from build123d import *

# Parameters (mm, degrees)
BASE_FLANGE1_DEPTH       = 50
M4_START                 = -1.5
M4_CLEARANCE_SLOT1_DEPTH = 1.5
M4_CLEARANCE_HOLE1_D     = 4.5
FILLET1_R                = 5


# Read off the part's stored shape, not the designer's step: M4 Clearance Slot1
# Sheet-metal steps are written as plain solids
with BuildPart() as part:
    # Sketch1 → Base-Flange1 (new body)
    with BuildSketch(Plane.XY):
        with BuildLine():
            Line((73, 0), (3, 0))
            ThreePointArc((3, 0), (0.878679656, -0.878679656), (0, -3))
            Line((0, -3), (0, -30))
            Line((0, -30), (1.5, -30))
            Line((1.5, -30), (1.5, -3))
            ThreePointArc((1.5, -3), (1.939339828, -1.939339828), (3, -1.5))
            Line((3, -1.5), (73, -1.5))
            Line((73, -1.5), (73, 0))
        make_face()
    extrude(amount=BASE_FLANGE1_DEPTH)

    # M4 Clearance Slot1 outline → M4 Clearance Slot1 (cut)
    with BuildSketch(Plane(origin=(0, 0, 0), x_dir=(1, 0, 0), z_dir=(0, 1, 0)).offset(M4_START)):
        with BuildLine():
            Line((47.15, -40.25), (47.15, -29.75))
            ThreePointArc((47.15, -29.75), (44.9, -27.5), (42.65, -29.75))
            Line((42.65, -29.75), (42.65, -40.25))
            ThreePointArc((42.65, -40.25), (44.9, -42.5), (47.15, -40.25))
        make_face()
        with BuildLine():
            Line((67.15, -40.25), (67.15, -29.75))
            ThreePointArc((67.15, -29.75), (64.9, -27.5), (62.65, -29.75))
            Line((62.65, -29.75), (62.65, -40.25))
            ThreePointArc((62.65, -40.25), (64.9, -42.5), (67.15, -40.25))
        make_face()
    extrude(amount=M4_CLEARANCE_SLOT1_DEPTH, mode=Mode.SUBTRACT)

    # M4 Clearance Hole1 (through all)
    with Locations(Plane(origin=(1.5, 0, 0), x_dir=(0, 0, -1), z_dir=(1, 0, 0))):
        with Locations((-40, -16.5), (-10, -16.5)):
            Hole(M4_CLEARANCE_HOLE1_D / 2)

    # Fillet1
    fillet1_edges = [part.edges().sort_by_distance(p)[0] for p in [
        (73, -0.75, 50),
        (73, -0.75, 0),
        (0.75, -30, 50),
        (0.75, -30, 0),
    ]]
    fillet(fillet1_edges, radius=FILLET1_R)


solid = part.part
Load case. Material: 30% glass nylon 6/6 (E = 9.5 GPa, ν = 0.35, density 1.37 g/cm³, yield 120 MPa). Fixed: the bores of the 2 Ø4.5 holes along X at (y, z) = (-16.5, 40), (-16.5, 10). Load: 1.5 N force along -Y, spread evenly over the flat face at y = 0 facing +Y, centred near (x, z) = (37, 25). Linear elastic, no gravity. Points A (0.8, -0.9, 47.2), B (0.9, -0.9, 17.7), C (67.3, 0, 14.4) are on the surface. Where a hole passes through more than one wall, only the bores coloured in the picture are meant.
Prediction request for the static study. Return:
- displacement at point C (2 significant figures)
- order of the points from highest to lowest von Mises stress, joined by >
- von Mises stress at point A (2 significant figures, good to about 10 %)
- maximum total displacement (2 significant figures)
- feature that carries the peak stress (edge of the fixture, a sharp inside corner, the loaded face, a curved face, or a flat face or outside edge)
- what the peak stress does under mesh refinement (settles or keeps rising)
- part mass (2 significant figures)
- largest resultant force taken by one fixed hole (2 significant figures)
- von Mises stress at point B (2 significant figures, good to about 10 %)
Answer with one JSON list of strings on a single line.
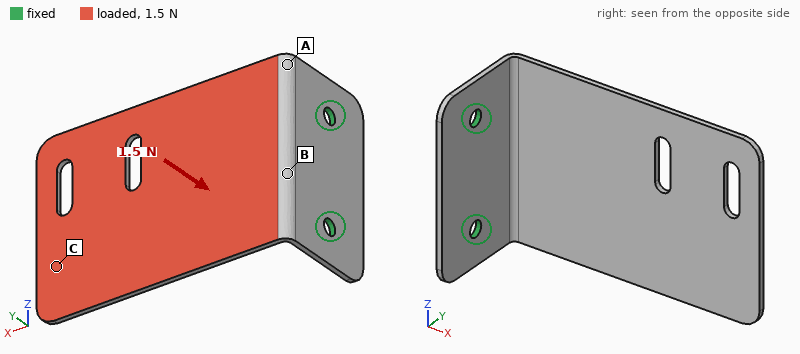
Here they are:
["0.81 mm", "B > A > C", "1.7 MPa", "0.89 mm", "edge of the fixture", "keeps rising", "10.0 g", "0.83 N", "2.2 MPa"]
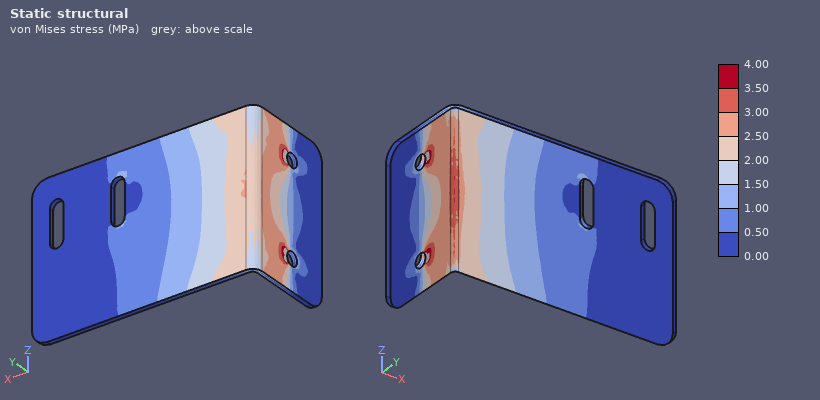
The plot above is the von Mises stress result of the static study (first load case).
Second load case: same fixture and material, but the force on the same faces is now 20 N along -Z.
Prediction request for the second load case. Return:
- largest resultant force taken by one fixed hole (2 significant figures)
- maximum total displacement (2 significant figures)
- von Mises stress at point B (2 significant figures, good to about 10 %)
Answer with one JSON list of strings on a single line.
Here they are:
["26 N", "1.00 mm", "8.0 MPa"]
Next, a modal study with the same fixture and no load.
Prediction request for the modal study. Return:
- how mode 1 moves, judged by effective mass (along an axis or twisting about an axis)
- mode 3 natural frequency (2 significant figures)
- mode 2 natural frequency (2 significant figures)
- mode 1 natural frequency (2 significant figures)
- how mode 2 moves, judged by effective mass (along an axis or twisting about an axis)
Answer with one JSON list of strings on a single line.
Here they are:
["along Y", "420 Hz", "300 Hz", "98 Hz", "along Z"]
